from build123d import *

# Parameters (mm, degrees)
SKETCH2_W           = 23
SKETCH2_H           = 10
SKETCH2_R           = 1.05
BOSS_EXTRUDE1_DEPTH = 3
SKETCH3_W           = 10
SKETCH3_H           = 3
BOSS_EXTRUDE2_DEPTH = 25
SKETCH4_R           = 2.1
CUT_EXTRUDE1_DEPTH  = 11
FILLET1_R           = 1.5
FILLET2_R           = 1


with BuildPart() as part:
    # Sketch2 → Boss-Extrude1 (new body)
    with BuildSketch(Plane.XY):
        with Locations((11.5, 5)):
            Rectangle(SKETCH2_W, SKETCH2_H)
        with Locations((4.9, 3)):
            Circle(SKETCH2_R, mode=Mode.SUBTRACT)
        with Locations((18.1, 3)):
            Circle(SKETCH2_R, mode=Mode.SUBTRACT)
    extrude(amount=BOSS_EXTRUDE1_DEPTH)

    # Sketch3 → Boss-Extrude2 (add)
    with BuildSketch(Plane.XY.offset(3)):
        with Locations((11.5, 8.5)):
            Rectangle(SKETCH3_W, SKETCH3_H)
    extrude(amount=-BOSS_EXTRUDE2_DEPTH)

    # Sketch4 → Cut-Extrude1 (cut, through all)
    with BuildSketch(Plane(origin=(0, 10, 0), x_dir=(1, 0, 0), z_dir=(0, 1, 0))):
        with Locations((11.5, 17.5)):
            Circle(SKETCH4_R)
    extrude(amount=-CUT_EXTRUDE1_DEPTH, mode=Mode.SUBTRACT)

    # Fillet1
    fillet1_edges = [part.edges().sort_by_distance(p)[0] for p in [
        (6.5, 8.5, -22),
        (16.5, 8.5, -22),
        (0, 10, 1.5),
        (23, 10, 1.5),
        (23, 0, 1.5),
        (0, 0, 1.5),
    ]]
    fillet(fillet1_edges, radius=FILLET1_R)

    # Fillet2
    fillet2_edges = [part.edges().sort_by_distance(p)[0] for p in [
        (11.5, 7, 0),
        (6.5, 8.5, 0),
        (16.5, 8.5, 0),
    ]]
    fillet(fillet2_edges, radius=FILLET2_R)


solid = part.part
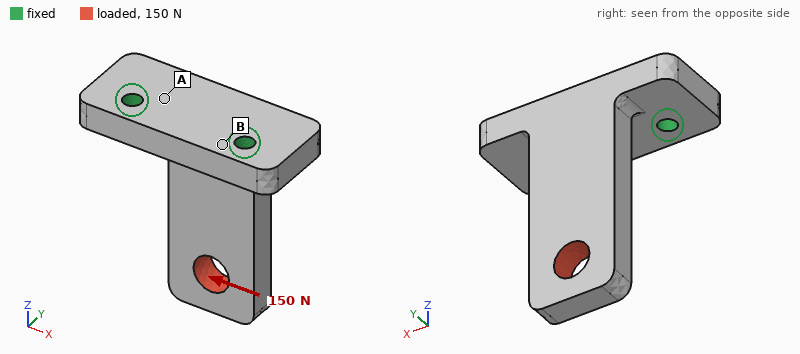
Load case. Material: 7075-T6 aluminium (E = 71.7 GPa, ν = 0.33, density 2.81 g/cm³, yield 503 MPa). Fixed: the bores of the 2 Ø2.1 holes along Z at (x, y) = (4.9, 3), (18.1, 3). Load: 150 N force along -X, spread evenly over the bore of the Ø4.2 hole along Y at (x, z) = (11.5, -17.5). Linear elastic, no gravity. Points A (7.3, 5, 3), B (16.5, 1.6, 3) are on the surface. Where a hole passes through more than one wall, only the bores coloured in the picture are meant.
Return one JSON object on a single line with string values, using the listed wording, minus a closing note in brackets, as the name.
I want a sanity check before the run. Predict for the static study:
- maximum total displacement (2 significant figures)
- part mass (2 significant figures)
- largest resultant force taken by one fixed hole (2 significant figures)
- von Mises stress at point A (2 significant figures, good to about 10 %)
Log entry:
{"maximum total displacement": "60 µm", "part mass": "3.6 g", "largest resultant force taken by one fixed hole": "240 N", "von Mises stress at point A": "22 MPa"}
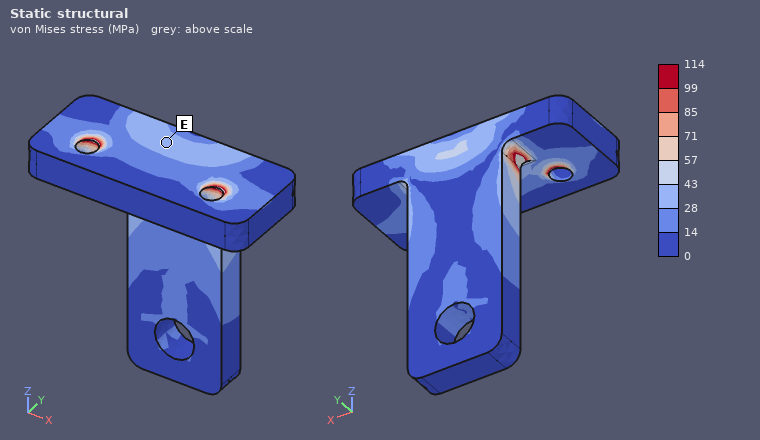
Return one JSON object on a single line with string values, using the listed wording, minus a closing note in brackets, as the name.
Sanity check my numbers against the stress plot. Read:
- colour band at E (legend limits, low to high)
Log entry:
{"colour band at E": "28 to 43 MPa"}
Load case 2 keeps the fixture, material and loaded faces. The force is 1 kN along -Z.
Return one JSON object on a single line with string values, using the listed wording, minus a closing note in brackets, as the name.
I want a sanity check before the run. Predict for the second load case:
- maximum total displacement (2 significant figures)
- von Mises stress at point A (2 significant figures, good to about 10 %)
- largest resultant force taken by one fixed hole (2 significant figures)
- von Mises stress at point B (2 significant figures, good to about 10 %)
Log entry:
{"maximum total displacement": "0.15 mm", "von Mises stress at point A": "97 MPa", "largest resultant force taken by one fixed hole": "500 N", "von Mises stress at point B": "76 MPa"}
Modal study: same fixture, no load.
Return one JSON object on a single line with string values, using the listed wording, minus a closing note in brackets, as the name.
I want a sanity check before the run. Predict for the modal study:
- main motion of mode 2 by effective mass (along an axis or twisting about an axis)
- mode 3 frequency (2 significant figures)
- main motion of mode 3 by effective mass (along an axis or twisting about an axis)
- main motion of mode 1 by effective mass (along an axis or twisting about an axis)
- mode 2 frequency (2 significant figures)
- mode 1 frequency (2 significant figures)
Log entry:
{"main motion of mode 2 by effective mass": "along X", "mode 3 frequency": "19 kHz", "main motion of mode 3 by effective mass": "along Z", "main motion of mode 1 by effective mass": "along Y", "mode 2 frequency": "9800 Hz", "mode 1 frequency": "4100 Hz"}
